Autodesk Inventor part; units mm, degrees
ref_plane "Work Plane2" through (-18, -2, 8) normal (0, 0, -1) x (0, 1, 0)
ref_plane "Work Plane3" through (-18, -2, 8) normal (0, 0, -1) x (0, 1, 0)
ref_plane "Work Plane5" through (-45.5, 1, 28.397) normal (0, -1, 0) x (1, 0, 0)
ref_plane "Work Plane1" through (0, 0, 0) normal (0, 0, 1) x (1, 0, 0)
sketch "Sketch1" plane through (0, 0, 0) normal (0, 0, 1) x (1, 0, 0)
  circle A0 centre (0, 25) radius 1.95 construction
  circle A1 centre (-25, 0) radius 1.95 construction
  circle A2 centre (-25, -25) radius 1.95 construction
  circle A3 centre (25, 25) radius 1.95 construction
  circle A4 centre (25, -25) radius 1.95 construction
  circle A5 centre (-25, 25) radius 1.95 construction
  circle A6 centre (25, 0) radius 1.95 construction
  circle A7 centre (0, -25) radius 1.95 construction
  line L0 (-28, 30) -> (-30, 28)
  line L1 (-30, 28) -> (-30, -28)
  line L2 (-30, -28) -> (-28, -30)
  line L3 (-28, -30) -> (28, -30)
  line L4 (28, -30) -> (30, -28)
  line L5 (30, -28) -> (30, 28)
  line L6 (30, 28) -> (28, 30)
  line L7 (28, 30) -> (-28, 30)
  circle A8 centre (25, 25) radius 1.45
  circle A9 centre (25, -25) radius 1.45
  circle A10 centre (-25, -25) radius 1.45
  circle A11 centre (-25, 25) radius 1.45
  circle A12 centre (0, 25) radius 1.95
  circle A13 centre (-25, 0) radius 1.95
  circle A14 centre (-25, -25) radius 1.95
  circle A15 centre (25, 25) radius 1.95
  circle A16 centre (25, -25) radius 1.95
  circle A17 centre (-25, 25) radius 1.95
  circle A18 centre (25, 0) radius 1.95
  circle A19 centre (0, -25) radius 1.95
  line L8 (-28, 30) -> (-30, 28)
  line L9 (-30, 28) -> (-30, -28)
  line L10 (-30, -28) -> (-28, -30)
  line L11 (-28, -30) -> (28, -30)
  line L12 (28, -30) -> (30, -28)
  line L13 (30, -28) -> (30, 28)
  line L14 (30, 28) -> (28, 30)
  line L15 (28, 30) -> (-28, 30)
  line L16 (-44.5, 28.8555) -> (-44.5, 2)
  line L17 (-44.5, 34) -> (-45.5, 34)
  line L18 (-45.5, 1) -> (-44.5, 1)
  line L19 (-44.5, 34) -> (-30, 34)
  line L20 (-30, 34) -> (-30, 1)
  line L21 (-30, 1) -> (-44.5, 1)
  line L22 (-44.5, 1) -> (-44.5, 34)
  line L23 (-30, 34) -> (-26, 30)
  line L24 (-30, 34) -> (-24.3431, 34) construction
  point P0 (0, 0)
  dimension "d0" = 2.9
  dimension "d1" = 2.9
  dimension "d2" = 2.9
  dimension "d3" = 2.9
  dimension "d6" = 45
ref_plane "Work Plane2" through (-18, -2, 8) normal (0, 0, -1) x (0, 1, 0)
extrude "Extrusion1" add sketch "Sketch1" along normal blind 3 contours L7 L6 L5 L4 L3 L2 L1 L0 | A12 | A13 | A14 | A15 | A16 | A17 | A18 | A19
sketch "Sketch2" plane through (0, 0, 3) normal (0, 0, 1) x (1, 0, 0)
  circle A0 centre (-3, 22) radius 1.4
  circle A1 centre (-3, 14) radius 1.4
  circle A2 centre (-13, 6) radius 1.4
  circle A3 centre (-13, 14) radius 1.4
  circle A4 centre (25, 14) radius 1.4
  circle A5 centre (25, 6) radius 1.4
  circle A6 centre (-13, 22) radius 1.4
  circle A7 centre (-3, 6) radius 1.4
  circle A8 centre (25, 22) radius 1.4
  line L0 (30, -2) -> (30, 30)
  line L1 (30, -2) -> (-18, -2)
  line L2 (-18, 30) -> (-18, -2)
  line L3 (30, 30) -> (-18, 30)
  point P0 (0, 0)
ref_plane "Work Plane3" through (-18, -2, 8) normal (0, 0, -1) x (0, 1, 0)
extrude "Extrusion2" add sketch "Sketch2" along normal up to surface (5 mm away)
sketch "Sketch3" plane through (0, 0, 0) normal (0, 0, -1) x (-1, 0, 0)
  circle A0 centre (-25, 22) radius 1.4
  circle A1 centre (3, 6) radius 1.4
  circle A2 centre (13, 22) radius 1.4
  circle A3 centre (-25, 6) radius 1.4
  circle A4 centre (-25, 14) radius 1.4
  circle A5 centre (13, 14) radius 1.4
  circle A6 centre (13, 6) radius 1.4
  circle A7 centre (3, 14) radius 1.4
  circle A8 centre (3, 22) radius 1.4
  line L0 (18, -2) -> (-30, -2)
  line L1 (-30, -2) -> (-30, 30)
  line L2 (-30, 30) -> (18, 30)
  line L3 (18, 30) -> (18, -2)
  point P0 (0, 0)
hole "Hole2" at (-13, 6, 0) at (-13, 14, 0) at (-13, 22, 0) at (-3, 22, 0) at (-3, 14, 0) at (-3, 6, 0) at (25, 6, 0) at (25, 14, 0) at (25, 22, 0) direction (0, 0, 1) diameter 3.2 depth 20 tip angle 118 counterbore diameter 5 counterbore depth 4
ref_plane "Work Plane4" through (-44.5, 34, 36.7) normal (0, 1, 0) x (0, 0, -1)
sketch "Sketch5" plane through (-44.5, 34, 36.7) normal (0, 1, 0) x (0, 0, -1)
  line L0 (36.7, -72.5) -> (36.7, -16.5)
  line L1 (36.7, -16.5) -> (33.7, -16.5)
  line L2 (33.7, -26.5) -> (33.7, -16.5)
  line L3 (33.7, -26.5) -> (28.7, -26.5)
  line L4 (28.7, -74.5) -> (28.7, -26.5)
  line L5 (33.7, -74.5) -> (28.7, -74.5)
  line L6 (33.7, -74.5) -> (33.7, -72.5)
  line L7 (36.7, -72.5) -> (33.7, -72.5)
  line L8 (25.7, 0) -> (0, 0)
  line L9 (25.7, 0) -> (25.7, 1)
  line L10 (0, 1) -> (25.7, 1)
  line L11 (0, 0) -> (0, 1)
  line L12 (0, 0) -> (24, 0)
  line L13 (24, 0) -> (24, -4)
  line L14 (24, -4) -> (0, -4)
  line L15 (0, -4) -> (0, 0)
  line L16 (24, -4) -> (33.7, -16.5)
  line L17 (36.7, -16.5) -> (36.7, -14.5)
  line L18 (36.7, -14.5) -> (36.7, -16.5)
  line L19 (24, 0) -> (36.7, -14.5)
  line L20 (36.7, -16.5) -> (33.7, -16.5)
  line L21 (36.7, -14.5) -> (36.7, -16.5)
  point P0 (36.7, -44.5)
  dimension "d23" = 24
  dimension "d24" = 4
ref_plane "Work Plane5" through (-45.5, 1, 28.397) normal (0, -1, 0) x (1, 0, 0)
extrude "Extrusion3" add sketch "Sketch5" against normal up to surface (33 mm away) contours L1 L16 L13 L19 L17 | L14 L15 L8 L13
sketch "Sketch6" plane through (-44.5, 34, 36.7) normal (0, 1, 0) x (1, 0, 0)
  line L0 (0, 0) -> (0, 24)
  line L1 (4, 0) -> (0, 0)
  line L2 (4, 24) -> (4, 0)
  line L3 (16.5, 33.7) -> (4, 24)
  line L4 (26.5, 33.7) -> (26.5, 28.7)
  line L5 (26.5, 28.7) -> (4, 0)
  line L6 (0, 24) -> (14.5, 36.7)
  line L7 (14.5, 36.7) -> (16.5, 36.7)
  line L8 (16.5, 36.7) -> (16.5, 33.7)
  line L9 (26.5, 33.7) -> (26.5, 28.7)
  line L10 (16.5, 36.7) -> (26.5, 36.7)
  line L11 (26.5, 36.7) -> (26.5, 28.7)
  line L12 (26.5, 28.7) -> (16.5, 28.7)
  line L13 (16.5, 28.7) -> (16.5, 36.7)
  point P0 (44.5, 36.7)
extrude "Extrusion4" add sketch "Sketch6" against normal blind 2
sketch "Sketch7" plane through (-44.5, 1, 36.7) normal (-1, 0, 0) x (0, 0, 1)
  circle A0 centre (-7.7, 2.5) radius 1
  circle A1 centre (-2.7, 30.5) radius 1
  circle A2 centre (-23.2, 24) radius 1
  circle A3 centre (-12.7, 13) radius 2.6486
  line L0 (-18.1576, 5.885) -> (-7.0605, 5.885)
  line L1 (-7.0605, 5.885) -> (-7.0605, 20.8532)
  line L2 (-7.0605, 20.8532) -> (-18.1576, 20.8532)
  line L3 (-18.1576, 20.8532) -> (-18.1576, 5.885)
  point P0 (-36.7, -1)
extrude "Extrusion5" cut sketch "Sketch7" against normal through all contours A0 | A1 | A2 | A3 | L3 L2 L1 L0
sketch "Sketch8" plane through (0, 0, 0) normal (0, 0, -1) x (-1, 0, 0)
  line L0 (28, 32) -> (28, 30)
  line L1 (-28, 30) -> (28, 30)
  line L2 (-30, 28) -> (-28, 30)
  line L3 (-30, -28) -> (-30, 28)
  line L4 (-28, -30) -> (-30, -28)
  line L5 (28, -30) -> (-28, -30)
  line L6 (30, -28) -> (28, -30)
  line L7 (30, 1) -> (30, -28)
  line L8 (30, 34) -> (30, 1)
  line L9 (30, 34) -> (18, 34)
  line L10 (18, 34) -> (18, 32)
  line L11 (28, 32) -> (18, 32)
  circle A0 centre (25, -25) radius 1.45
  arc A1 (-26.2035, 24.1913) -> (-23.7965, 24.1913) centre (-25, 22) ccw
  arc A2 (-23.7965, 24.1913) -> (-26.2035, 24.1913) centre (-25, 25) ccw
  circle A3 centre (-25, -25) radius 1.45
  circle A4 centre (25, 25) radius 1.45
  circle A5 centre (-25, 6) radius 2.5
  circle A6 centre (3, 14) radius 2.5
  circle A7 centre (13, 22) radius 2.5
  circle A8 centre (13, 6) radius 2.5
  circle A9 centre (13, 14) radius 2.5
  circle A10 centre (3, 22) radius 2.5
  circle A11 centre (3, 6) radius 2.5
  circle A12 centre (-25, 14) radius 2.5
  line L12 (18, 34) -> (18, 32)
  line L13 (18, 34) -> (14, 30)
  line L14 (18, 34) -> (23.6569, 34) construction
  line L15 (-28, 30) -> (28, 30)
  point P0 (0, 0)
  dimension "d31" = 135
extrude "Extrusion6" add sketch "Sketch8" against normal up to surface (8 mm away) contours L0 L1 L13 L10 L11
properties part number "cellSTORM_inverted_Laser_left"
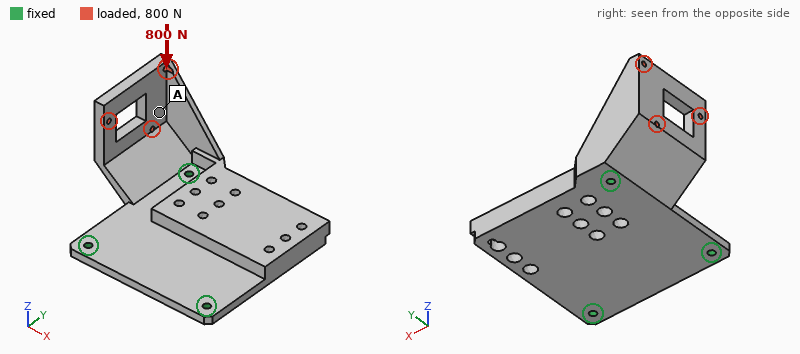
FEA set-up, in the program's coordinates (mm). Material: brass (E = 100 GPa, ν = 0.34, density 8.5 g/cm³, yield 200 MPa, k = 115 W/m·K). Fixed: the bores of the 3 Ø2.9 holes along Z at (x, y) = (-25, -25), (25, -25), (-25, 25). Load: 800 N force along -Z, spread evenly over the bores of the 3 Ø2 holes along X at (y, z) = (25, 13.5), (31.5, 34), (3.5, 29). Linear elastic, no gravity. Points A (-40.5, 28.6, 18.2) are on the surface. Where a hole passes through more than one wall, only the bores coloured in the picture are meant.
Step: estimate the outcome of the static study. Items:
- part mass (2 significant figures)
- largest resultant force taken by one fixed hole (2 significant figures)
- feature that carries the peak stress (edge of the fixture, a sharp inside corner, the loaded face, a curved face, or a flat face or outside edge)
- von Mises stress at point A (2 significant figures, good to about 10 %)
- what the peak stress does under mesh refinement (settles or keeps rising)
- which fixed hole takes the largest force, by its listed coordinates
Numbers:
190 g
880 N
edge of the fixture
21 MPa
keeps rising
(-25, 25)
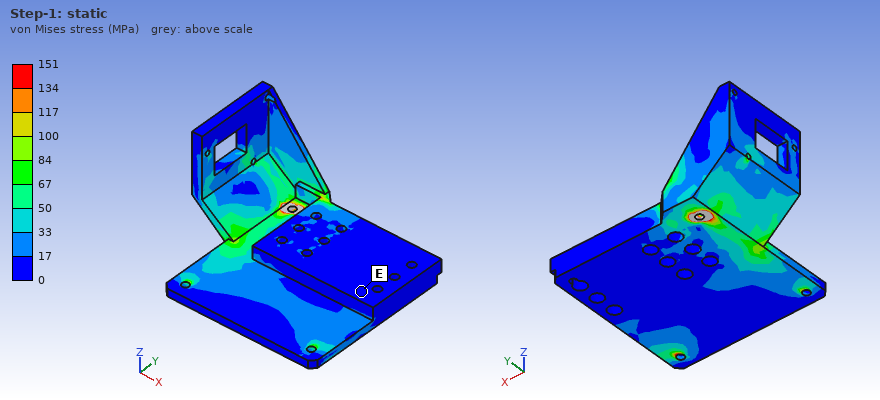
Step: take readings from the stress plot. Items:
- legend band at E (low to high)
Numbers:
0 to 17 MPa
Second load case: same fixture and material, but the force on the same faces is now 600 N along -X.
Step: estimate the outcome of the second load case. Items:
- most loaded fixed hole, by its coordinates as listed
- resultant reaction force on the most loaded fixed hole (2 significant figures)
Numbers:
(25, -25)
570 N
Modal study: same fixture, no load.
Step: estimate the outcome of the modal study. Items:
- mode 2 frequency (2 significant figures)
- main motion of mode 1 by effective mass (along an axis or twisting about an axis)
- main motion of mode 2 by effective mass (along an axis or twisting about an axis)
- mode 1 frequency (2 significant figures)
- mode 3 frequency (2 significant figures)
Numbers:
1500 Hz
along Z
along Z
1000 Hz
1900 Hz
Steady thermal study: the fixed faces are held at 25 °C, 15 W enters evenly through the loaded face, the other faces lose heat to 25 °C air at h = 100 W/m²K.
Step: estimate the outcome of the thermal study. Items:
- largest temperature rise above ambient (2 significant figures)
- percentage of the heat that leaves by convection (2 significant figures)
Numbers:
32 K
53 %
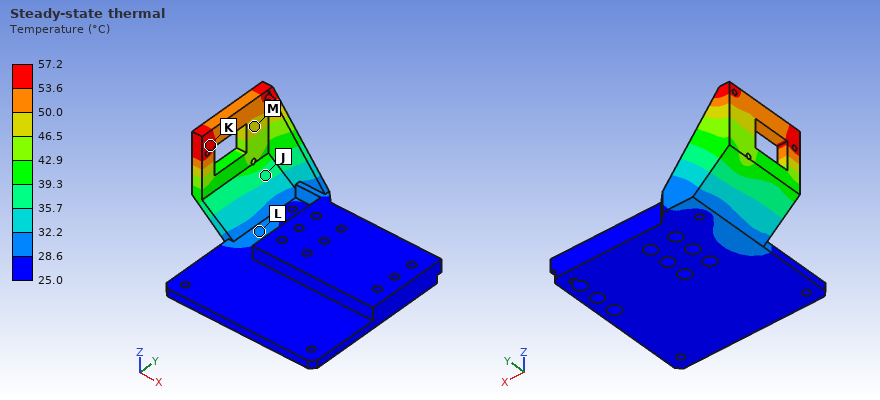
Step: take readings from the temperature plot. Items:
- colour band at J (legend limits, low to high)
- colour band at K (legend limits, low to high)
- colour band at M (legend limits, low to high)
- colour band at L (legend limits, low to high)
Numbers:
35.7 to 39.3 °C
53.6 to 57.2 °C
46.5 to 50.0 °C
28.6 to 32.2 °C
